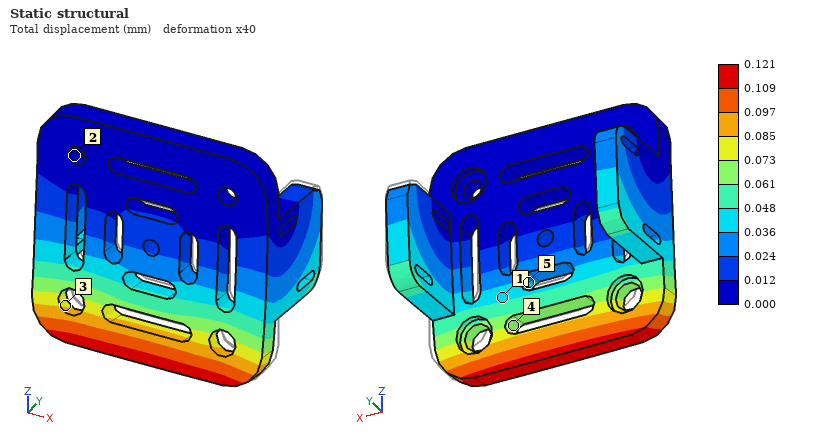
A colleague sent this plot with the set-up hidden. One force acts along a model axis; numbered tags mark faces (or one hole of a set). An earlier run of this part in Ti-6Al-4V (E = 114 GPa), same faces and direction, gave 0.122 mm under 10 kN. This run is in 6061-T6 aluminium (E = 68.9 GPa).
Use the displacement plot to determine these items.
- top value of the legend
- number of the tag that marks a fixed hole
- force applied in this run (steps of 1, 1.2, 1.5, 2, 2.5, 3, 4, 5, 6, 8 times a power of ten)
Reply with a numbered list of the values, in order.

1. 0.121 mm
2. 2
3. 6 kN
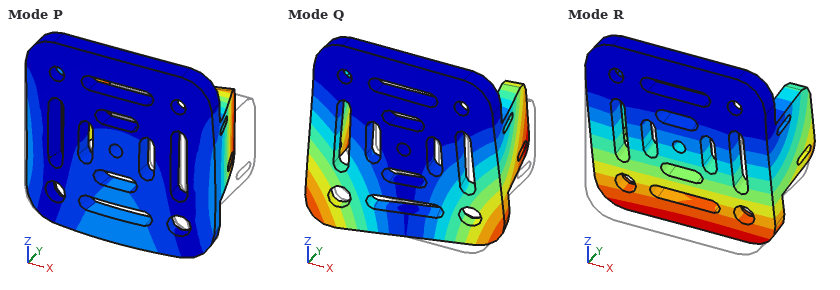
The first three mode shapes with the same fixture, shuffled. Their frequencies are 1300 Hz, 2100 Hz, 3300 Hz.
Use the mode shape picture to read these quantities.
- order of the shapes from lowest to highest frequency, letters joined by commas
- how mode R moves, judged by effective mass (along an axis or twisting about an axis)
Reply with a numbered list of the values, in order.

1. R, Q, P
2. along Y
